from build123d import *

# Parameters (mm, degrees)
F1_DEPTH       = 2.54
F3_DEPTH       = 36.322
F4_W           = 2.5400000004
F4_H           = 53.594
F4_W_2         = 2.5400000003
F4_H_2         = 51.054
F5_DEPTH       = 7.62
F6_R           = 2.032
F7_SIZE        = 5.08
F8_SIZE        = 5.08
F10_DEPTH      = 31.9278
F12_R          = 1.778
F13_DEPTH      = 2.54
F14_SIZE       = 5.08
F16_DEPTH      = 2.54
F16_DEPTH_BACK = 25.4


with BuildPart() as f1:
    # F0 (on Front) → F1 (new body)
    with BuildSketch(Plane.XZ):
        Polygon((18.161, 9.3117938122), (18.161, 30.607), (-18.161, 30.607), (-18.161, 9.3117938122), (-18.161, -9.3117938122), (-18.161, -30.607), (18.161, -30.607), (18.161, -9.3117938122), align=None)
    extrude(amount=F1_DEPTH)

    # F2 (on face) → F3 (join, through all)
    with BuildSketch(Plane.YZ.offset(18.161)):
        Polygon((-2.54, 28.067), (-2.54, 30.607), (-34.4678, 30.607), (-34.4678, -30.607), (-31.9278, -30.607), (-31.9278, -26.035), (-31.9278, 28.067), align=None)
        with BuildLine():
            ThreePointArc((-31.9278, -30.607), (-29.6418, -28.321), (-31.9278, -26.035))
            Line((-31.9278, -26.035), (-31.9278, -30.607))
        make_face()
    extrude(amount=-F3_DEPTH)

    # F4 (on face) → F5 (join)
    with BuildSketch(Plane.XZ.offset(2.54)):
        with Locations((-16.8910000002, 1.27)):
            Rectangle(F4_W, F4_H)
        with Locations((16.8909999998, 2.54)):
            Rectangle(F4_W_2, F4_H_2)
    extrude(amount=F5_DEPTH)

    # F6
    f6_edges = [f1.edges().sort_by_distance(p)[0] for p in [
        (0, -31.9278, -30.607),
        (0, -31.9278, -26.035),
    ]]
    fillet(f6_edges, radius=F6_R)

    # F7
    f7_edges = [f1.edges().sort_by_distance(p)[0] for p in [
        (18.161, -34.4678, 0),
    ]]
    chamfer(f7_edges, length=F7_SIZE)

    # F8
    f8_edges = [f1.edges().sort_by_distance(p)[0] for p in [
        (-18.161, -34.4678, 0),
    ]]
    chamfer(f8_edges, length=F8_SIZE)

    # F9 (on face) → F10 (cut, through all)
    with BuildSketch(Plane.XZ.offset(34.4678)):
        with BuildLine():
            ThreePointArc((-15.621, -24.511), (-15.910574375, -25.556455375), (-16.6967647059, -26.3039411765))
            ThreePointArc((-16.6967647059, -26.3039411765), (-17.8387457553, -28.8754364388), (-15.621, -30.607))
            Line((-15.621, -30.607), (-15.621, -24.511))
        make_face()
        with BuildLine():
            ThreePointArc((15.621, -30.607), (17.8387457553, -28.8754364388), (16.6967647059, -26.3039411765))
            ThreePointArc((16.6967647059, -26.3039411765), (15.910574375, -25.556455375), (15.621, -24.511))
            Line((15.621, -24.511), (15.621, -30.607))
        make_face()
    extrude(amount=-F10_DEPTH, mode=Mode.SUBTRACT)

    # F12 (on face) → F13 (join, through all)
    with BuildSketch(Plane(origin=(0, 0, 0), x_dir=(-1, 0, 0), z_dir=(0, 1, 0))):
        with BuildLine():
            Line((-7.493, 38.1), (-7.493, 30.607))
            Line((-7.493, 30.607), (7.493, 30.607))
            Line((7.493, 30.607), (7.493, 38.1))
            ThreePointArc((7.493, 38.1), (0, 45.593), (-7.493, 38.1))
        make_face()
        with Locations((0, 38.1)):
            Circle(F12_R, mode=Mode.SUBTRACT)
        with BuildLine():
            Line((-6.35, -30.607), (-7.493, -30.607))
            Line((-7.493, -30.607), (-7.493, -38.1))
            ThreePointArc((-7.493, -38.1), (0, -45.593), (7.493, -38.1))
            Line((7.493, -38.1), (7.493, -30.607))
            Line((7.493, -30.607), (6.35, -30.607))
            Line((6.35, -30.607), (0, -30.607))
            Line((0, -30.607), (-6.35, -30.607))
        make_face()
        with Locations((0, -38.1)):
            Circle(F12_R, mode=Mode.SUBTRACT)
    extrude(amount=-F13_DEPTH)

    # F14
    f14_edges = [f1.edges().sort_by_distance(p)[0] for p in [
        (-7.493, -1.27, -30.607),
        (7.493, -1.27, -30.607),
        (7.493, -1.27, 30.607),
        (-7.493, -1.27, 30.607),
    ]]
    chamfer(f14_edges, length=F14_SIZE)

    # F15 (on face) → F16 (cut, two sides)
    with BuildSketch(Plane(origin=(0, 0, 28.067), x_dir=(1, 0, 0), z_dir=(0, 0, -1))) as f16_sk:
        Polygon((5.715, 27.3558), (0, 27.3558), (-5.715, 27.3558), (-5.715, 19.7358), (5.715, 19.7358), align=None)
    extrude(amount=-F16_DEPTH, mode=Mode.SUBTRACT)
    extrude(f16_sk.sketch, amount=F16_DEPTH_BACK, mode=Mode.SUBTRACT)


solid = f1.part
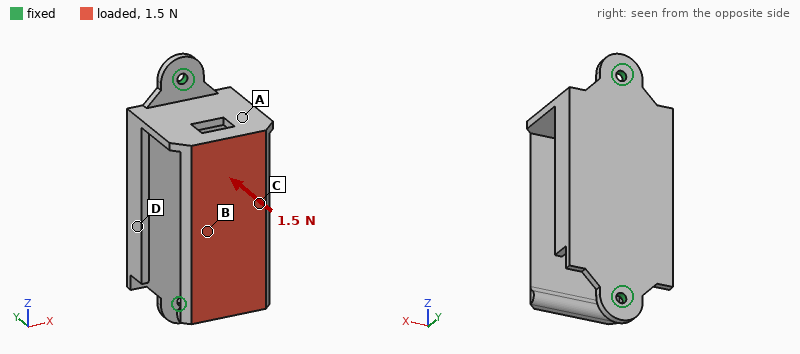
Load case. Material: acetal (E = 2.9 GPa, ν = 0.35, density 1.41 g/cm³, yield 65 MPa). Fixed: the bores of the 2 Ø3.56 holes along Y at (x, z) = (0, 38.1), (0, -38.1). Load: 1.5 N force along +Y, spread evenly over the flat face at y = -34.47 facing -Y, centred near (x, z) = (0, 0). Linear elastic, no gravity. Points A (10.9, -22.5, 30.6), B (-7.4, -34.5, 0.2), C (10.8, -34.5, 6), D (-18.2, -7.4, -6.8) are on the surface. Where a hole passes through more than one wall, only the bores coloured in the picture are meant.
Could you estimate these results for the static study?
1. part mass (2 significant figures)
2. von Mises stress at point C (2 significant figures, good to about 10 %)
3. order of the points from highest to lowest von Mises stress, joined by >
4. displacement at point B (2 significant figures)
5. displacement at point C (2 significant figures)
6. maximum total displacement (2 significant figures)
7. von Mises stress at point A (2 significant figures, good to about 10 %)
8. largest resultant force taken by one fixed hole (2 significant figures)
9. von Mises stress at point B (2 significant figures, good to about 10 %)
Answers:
23 g
0.56 MPa
A > C > B > D
0.46 mm
0.37 mm
1.0 mm
1.6 MPa
1.3 N
0.40 MPa
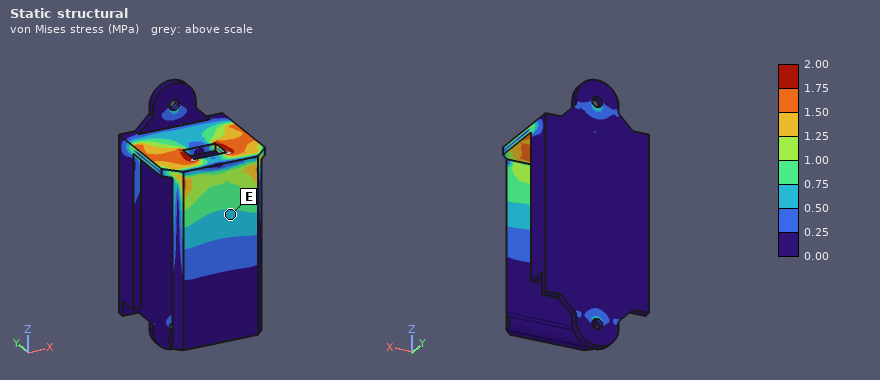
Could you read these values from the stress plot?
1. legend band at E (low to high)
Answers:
0.50 to 0.75 MPa
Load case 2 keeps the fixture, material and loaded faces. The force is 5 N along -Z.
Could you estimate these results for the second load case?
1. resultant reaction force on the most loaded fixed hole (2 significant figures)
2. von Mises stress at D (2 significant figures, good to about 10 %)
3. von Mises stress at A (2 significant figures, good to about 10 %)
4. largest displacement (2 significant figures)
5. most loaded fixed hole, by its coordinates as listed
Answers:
5.1 N
0.30 MPa
2.3 MPa
1.2 mm
(0, -38.1)
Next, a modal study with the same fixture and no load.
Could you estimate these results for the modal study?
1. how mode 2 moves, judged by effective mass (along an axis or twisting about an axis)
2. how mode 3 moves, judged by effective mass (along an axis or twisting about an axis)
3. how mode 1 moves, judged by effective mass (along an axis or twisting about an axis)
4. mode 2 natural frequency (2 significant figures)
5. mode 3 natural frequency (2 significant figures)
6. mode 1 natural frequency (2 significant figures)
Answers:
along X
along Z
along Y
150 Hz
320 Hz
86 Hz
